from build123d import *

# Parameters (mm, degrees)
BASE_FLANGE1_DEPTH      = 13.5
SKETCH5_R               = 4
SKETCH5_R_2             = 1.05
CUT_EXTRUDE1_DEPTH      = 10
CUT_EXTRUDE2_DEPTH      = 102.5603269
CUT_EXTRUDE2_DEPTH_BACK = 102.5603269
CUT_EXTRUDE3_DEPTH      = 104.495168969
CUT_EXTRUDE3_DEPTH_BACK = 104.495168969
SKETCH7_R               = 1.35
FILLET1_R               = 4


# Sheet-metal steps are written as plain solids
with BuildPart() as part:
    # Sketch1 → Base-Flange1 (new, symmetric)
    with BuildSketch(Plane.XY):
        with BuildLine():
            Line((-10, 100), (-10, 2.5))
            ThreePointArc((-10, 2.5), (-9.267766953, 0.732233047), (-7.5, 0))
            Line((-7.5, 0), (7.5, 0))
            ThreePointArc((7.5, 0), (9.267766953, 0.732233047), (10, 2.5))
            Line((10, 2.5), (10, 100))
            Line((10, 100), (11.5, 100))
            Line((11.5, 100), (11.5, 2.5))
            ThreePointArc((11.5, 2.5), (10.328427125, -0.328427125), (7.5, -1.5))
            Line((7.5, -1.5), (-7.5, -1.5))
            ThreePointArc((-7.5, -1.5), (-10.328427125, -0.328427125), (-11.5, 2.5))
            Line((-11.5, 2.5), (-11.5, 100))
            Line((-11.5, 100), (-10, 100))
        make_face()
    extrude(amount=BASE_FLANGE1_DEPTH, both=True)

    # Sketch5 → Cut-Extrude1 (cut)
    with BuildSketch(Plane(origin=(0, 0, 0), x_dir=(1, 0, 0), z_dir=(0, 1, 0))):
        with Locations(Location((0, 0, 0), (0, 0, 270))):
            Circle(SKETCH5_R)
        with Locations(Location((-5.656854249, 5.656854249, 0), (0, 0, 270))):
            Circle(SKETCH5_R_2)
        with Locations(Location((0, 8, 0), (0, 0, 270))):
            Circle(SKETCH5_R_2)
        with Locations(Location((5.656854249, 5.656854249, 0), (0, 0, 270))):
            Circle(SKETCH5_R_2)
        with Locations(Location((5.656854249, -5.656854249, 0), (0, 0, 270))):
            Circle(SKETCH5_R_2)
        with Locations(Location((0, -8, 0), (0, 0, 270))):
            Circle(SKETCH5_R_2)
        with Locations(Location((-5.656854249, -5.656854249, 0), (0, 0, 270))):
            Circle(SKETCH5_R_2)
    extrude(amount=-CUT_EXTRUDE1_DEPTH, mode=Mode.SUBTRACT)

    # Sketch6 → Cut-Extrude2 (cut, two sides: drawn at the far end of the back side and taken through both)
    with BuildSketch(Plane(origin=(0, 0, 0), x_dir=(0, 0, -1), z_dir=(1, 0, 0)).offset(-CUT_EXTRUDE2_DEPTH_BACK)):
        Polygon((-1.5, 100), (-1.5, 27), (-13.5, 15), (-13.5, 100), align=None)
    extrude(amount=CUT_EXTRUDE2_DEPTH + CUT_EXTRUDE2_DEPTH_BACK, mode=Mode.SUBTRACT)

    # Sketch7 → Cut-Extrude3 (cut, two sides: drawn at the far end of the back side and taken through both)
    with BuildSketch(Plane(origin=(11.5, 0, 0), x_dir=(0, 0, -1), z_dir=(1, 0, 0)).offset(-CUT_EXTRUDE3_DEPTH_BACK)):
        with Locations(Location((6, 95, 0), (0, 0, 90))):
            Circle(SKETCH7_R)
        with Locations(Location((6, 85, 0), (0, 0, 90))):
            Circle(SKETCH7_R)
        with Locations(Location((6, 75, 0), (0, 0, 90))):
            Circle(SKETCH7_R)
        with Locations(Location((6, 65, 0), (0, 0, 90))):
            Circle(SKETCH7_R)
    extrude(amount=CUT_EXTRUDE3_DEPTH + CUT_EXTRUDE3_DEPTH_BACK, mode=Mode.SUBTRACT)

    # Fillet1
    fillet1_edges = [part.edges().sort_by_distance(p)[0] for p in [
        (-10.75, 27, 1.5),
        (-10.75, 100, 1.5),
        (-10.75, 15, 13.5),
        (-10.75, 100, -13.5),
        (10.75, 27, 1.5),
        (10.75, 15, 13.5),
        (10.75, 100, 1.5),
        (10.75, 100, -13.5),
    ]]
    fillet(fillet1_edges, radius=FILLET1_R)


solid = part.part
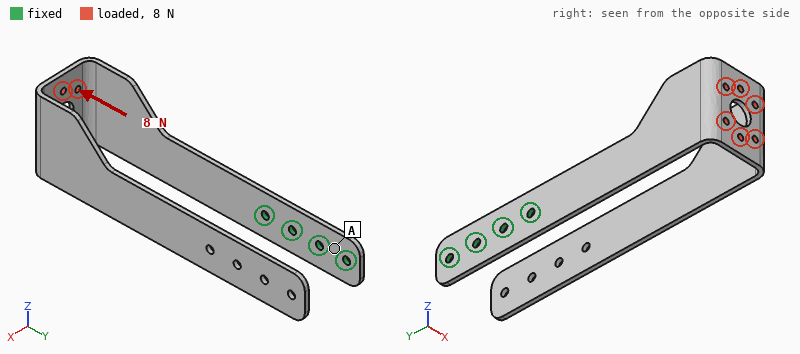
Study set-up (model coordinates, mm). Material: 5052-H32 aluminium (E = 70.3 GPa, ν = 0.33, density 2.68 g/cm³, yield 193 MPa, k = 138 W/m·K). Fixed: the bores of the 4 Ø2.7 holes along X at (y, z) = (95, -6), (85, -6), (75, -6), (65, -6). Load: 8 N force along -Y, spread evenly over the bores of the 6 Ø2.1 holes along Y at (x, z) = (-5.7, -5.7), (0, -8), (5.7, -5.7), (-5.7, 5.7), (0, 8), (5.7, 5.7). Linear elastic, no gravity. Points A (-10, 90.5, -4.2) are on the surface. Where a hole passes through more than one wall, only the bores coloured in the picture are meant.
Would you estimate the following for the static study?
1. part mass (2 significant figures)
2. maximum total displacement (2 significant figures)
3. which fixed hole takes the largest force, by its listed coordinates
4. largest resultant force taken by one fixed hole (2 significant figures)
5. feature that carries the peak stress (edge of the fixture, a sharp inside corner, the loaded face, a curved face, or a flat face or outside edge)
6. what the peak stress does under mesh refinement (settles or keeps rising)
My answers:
16 g
1.2 mm
(65, -6)
7.0 N
edge of the fixture
keeps rising
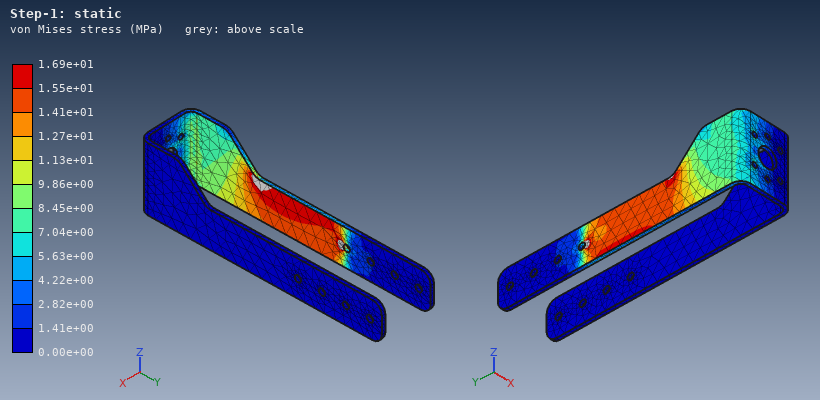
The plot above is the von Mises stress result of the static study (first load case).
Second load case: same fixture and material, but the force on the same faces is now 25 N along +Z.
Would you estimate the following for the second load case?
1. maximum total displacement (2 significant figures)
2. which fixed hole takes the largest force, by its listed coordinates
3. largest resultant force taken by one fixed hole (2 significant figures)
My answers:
1.1 mm
(65, -6)
120 N
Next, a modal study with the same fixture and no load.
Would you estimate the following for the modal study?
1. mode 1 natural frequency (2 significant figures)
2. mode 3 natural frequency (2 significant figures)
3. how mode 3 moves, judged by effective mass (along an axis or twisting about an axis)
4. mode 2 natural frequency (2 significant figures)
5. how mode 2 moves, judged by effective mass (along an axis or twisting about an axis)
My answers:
81 Hz
160 Hz
along Z
130 Hz
along X
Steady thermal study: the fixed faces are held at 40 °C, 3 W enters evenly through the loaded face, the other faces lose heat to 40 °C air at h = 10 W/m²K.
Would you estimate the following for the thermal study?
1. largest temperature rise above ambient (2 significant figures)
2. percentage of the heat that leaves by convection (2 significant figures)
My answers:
31 K
55 %
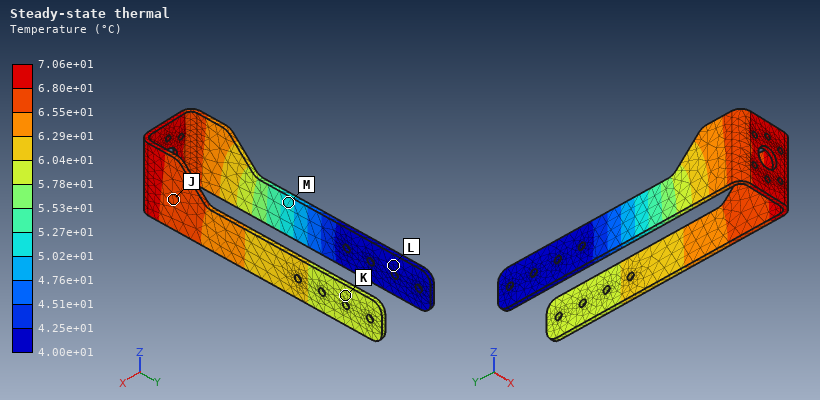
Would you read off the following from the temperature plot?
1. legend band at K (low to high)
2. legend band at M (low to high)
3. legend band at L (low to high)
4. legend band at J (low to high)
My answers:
5.78e+01 to 6.04e+01 °C
5.02e+01 to 5.27e+01 °C
4.00e+01 to 4.25e+01 °C
6.55e+01 to 6.80e+01 °C
